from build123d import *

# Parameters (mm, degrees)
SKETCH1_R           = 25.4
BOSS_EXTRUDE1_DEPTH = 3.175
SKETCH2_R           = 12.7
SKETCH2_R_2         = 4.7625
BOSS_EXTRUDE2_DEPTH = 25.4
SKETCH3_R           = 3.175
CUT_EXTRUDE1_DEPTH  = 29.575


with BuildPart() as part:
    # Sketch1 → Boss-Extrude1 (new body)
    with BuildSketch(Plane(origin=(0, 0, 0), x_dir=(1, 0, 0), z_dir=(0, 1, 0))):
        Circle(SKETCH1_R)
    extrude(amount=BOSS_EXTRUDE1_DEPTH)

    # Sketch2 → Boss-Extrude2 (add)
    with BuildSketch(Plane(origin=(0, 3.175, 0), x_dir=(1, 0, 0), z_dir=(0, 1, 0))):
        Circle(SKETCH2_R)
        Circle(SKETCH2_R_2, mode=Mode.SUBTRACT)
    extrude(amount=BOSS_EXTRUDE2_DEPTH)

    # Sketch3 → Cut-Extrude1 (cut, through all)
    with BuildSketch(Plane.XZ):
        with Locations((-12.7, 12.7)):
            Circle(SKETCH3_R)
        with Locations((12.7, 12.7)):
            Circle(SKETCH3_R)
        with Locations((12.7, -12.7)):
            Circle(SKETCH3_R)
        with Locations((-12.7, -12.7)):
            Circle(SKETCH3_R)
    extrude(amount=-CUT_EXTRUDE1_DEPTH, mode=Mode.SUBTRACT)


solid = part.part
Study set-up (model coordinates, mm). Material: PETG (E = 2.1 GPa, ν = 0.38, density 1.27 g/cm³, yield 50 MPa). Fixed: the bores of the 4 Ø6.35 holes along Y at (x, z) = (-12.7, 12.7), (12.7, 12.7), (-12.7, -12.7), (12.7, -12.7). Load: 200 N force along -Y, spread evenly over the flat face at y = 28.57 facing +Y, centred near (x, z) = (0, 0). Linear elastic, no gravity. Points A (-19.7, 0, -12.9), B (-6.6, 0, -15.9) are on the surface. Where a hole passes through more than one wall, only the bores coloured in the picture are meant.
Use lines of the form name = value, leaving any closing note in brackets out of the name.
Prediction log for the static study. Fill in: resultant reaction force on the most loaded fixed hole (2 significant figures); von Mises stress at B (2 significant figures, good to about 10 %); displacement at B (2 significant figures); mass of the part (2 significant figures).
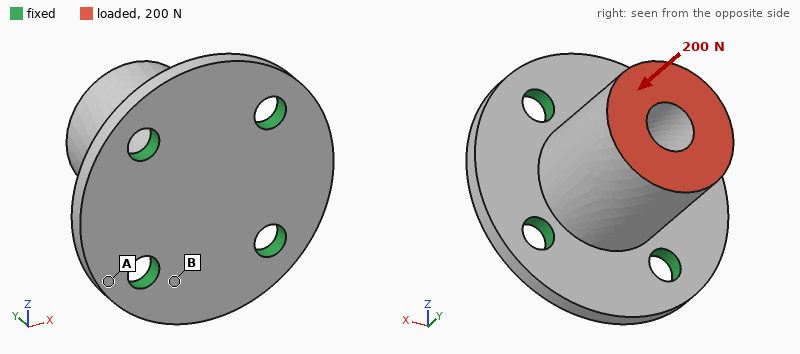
resultant reaction force on the most loaded fixed hole = 54 N
von Mises stress at B = 0.80 MPa
displacement at B = 5.3 µm
mass of the part = 22 g
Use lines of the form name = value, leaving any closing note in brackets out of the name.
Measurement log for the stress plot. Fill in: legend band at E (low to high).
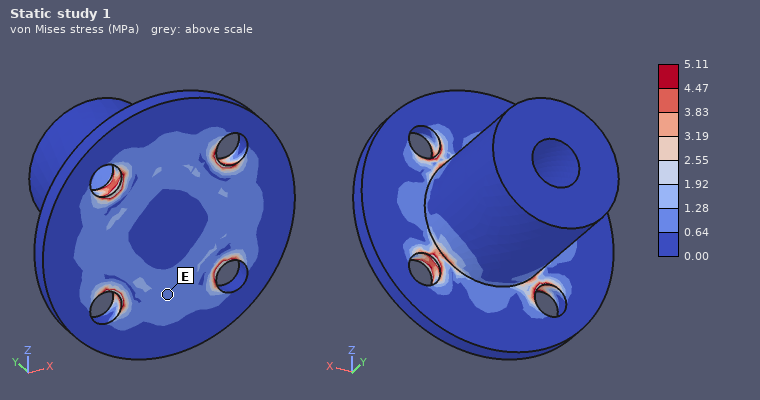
legend band at E = 0.64 to 1.28 MPa
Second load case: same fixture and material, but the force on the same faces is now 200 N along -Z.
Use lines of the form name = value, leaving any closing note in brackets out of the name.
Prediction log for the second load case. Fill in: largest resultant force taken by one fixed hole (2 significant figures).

largest resultant force taken by one fixed hole = 140 N
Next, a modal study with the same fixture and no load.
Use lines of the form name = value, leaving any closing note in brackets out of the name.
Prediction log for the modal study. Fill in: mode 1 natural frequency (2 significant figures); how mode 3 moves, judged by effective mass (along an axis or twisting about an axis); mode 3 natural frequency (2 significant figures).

mode 1 natural frequency = 2600 Hz
how mode 3 moves, judged by effective mass = along Y
mode 3 natural frequency = 4300 Hz
